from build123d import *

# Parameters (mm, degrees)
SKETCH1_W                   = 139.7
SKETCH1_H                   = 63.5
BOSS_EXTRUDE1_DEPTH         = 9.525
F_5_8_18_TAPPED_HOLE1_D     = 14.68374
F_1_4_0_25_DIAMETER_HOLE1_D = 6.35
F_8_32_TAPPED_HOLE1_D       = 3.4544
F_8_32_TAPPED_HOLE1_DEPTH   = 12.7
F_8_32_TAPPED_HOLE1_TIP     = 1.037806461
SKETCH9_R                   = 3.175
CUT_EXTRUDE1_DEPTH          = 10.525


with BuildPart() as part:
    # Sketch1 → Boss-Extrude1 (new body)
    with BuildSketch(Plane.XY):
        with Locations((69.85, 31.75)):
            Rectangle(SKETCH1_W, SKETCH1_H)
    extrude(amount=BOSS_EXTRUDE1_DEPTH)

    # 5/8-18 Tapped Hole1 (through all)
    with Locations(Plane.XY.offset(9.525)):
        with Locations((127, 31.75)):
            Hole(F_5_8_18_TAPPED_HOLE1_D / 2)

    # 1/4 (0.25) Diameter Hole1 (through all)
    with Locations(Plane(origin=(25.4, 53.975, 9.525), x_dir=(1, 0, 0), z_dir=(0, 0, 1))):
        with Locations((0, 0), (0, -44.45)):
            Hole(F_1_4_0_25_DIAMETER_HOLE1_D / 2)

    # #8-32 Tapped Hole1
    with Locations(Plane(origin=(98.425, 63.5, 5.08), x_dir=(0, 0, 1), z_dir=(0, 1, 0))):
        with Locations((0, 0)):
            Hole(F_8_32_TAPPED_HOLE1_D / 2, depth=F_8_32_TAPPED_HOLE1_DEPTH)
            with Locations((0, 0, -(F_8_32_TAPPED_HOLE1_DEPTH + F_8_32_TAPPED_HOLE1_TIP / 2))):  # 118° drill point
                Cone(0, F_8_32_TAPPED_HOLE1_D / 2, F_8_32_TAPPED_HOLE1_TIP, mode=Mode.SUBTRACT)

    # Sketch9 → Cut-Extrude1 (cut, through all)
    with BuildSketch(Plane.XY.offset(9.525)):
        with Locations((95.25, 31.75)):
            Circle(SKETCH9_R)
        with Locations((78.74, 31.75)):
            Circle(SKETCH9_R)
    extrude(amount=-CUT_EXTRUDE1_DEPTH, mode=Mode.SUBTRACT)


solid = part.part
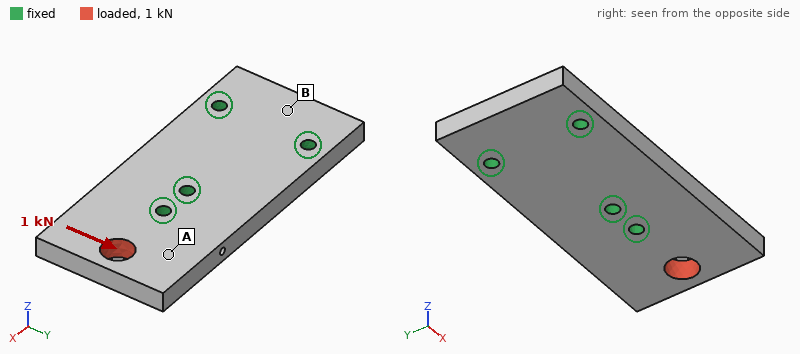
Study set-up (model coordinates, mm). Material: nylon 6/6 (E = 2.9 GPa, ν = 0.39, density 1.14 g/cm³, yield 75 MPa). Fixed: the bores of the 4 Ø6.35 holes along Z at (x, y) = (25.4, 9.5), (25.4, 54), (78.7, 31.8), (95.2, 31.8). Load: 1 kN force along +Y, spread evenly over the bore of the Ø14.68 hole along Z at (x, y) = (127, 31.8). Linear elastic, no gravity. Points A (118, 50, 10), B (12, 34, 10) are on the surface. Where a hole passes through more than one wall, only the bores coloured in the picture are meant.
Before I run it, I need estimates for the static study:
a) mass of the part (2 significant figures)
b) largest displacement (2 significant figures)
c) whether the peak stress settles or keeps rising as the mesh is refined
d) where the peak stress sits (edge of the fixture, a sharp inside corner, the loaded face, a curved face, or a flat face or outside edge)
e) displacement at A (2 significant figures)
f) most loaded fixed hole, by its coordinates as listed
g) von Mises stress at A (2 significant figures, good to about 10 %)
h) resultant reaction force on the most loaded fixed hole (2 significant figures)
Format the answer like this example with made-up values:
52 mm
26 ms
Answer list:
93 g
0.24 mm
keeps rising
edge of the fixture
0.12 mm
(95.2, 31.8)
2.8 MPa
1.4 kN
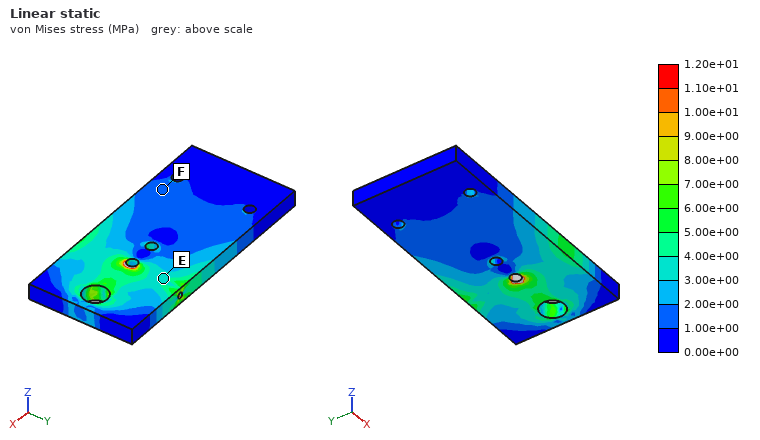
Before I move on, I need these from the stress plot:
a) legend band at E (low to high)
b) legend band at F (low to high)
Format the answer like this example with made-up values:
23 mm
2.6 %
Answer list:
3.00e+00 to 4.00e+00 MPa
1.00e+00 to 2.00e+00 MPa
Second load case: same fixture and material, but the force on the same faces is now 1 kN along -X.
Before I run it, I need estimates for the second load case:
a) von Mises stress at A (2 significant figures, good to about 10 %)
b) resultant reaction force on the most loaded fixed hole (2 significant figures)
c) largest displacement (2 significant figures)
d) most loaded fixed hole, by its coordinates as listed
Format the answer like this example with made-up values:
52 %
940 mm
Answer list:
1.6 MPa
620 N
71 µm
(95.2, 31.8)
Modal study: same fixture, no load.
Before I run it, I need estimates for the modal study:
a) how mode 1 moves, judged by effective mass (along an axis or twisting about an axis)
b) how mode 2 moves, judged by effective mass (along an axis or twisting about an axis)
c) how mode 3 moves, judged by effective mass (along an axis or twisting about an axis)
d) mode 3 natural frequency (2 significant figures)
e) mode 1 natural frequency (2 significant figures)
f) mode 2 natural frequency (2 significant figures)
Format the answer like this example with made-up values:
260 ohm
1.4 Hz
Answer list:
along Z
twisting about X
along Y
2700 Hz
1100 Hz
1300 Hz
